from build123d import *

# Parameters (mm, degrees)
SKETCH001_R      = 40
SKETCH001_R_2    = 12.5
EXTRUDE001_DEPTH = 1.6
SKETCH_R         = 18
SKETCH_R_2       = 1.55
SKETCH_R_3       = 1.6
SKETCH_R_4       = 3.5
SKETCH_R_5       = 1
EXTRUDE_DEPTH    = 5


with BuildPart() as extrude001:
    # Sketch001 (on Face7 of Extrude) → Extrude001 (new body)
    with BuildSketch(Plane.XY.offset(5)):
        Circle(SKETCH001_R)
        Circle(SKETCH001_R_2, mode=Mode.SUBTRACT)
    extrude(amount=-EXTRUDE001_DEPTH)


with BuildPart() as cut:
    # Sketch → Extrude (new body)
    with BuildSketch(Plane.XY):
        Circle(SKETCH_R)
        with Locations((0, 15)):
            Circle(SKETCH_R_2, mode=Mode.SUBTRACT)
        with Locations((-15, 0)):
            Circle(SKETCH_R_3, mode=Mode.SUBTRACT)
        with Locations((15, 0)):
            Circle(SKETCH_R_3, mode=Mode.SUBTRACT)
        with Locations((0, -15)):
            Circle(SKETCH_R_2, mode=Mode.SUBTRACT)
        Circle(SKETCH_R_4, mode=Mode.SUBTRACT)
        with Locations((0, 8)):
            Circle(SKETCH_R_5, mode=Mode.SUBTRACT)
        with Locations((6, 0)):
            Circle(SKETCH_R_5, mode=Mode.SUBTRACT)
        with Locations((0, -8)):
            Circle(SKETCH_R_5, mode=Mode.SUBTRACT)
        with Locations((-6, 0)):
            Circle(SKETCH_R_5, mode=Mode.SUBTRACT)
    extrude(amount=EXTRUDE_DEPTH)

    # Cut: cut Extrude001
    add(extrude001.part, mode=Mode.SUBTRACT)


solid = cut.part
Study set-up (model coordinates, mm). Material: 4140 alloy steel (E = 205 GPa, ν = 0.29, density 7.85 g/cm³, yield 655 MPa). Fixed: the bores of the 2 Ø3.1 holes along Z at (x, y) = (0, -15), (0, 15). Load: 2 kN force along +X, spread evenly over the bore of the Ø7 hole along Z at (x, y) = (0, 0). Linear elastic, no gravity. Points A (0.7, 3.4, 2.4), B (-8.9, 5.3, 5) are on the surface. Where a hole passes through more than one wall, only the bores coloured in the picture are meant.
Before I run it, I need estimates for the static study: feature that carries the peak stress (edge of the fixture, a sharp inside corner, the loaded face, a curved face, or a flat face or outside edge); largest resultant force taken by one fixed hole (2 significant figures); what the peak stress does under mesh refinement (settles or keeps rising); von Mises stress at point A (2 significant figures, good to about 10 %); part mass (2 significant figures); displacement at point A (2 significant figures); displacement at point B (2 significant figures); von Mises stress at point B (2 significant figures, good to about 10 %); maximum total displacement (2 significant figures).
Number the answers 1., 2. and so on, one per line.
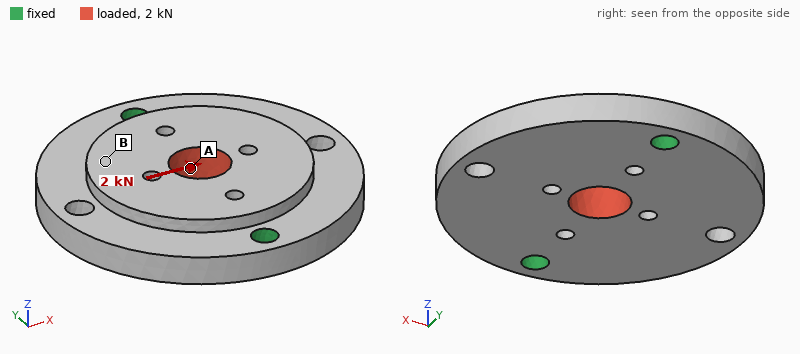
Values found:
1. edge of the fixture
2. 1.0 kN
3. keeps rising
4. 32 MPa
5. 30 g
6. 2.5 µm
7. 3.4 µm
8. 13 MPa
9. 5.0 µm
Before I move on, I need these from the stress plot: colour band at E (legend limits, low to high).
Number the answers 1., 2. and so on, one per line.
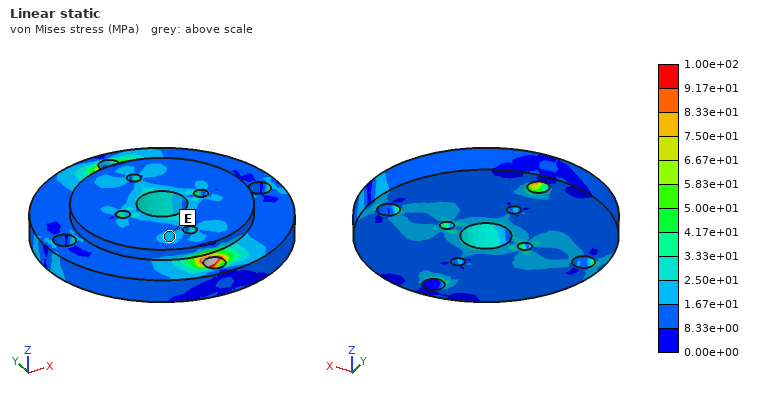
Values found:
1. 1.67e+01 to 2.50e+01 MPa
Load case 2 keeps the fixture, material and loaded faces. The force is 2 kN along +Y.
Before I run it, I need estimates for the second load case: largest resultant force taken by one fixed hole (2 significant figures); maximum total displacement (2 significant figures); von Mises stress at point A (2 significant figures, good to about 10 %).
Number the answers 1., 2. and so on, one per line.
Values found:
1. 1.0 kN
2. 1.7 µm
3. 18 MPa
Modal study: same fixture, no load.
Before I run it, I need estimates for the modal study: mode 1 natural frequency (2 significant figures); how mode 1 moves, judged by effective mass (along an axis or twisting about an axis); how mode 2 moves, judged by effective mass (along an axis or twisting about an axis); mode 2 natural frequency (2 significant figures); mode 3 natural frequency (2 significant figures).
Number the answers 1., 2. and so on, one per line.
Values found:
1. 8000 Hz
2. twisting about Y
3. along Z
4. 12 kHz
5. 24 kHz
